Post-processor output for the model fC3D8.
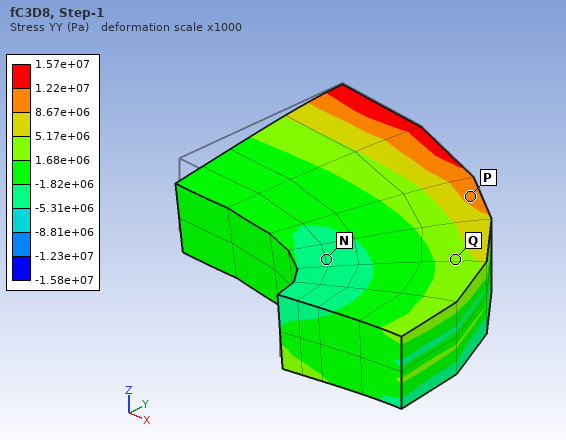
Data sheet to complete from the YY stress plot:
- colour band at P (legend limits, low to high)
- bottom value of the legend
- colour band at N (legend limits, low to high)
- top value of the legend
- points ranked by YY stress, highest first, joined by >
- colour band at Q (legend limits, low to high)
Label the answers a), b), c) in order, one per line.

a) 8.67e+06 to 1.22e+07 Pa
b) -1.58e+07 Pa
c) -5.31e+06 to -1.82e+06 Pa
d) 1.57e+07 Pa
e) P > Q > N
f) 1.68e+06 to 5.17e+06 Pa
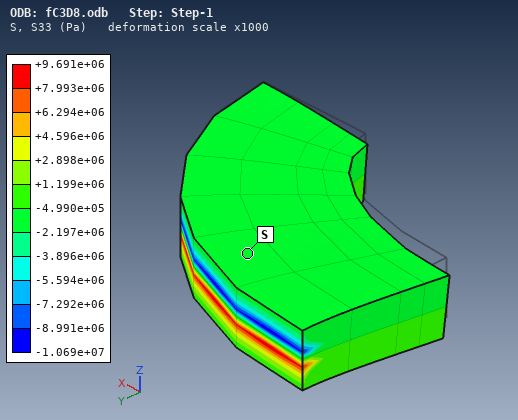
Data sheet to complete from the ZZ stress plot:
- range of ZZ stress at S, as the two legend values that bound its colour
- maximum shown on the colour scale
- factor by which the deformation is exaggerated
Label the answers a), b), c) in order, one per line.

a) -2.197e+06 to -4.990e+05 Pa
b) +9.691e+06 Pa
c) 1000
